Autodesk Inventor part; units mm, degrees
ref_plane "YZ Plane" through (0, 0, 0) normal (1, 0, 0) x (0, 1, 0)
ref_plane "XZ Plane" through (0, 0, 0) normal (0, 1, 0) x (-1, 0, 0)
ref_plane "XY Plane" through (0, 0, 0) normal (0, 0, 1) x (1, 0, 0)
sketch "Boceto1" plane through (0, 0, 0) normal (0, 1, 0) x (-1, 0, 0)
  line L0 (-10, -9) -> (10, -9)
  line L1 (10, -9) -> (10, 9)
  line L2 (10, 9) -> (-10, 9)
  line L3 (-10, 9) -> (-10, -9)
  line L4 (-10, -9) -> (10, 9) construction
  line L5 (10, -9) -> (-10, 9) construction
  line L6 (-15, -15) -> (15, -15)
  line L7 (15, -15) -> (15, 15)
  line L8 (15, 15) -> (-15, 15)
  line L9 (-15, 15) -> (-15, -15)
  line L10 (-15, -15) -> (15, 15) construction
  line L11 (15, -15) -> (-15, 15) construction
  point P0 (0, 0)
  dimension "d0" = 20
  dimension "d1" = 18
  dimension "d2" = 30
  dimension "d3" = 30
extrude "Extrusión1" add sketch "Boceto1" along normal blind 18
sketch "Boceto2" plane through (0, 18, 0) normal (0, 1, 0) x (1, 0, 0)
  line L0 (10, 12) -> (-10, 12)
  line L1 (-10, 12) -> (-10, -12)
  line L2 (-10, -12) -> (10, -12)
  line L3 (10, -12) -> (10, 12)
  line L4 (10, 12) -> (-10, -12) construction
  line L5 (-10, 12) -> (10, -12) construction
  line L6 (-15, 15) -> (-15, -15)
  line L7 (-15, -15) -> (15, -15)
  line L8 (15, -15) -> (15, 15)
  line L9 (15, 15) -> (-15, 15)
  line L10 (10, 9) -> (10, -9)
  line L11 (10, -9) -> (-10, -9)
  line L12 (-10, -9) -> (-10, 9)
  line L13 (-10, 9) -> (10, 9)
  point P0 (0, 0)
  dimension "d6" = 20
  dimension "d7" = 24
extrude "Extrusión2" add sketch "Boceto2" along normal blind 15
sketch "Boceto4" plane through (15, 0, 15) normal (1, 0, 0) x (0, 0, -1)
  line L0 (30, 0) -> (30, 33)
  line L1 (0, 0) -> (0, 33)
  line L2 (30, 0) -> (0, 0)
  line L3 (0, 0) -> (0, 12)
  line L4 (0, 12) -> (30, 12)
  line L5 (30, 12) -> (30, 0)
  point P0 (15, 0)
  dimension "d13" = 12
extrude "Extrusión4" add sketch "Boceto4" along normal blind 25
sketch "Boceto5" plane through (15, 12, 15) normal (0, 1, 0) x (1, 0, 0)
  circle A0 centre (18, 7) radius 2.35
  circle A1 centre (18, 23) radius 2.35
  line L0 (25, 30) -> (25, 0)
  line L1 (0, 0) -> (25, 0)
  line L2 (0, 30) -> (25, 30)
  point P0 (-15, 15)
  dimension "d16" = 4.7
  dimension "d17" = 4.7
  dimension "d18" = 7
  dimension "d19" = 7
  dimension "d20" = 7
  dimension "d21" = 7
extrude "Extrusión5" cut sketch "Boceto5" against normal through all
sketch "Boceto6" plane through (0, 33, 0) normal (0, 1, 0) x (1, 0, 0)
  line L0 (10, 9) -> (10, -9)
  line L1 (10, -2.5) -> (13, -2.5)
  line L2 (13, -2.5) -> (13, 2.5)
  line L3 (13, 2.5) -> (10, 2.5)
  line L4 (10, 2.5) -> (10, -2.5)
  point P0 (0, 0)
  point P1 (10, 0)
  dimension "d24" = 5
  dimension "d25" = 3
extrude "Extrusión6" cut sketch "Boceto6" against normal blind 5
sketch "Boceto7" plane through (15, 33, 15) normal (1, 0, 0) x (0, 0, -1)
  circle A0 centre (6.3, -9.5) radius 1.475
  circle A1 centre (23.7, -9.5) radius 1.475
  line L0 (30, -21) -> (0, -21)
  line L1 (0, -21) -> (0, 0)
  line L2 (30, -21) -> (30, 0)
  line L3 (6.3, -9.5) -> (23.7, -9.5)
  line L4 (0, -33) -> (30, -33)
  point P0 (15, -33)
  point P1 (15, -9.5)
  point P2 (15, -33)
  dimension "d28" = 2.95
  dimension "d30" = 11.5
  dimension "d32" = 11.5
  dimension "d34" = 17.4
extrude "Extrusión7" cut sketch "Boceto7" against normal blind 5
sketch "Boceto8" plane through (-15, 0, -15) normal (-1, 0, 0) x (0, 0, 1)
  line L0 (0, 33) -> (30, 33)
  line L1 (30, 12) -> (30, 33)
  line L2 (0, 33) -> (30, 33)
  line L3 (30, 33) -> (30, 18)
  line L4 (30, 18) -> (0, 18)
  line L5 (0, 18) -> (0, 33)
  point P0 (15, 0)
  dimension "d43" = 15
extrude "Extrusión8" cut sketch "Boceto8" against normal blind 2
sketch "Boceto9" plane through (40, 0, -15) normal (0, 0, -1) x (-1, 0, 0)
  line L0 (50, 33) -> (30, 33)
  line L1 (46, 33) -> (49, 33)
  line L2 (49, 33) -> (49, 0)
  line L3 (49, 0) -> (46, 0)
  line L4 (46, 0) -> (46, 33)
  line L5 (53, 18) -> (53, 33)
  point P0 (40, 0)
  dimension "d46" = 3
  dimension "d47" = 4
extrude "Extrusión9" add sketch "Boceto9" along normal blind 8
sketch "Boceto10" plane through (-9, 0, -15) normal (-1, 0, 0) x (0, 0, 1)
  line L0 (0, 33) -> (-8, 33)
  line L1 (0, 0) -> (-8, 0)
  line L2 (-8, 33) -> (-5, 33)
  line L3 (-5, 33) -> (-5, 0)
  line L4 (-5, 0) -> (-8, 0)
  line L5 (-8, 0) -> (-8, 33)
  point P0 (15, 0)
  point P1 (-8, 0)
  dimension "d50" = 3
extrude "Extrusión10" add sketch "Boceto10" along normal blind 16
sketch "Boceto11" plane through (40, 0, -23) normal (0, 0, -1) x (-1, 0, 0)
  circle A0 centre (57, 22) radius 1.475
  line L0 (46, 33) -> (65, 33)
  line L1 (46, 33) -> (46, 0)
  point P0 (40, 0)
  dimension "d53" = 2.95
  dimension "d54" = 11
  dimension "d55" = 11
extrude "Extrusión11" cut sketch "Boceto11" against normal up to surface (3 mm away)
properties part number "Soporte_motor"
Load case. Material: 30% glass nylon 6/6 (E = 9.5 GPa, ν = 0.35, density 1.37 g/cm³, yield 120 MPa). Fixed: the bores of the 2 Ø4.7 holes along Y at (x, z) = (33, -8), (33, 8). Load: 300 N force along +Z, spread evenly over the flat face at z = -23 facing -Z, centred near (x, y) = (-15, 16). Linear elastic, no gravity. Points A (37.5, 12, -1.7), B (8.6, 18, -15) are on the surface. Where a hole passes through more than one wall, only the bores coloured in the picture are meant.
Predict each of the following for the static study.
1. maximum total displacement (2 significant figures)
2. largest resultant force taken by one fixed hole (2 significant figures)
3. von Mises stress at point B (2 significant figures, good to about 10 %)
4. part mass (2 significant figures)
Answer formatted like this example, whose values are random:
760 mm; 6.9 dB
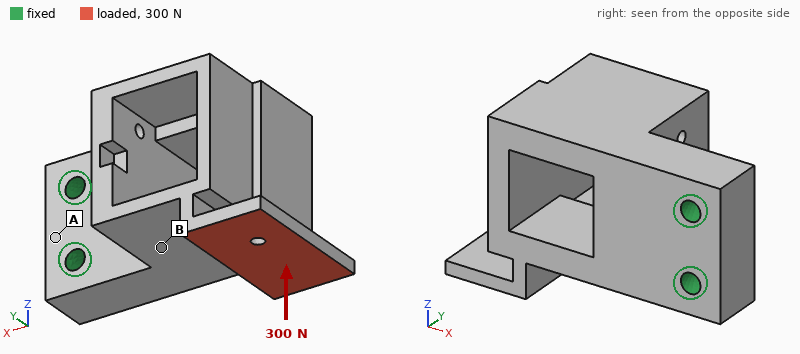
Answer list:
0.90 mm; 780 N; 9.3 MPa; 36 g
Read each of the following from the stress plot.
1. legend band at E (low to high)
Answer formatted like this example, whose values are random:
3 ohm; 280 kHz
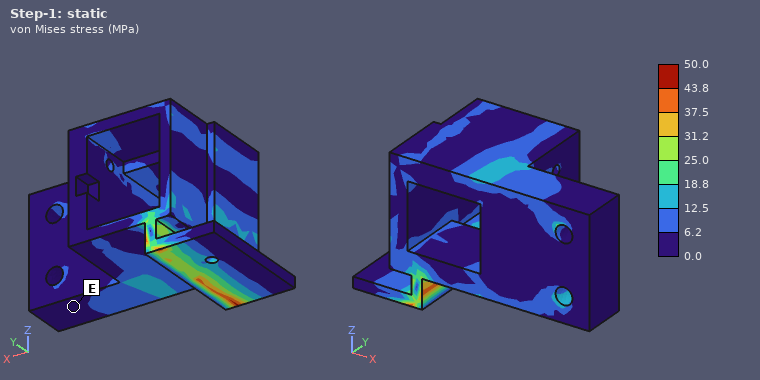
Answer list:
0.0 to 6.2 MPa
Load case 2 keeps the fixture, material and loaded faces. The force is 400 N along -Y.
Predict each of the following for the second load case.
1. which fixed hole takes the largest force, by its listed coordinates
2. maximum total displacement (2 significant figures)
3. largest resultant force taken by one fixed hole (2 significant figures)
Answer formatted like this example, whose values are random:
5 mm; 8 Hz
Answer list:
(33, -8); 0.94 mm; 550 N
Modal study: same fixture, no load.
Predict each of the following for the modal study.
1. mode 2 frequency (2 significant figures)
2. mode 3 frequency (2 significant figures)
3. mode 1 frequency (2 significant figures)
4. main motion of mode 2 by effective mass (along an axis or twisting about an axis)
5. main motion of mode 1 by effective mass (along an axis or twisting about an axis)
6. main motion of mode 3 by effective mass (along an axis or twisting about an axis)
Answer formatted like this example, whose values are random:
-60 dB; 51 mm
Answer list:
1800 Hz; 2500 Hz; 1300 Hz; along Z; along Y; twisting about X
